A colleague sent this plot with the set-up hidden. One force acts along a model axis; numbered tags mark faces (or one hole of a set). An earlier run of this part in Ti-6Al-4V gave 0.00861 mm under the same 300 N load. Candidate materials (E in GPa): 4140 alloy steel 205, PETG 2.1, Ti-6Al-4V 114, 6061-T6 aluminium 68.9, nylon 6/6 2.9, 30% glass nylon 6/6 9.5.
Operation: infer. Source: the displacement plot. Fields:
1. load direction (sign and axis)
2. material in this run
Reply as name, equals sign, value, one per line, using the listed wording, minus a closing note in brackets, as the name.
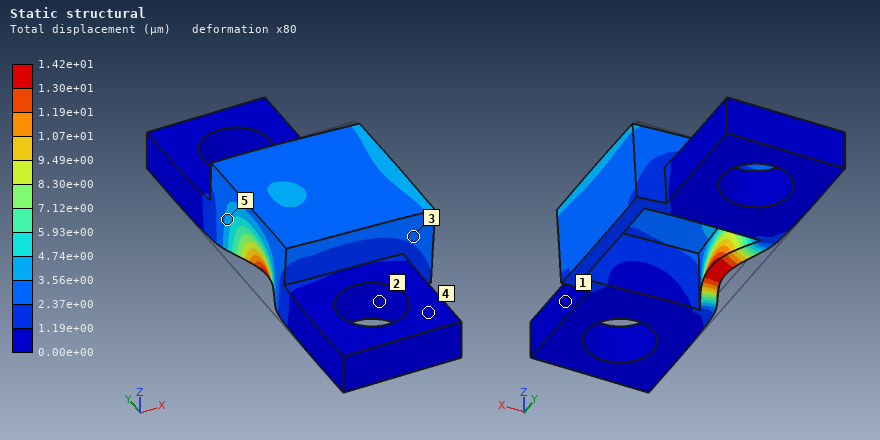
load direction = +X
material in this run = 6061-T6 aluminium
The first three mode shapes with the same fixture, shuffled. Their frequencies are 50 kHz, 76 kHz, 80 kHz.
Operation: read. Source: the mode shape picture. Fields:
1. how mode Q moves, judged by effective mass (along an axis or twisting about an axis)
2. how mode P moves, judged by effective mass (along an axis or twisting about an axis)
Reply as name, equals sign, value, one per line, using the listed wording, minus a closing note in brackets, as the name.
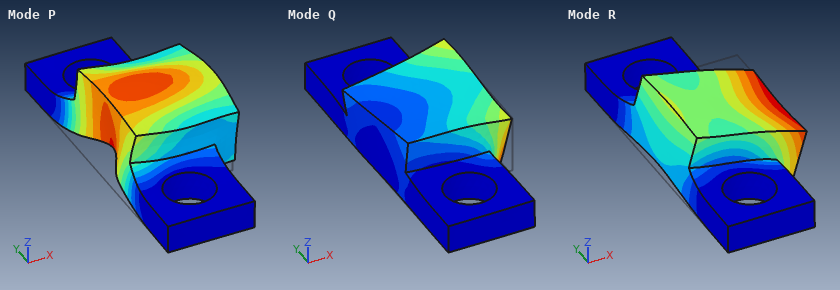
how mode Q moves, judged by effective mass = along Y
how mode P moves, judged by effective mass = along Z
